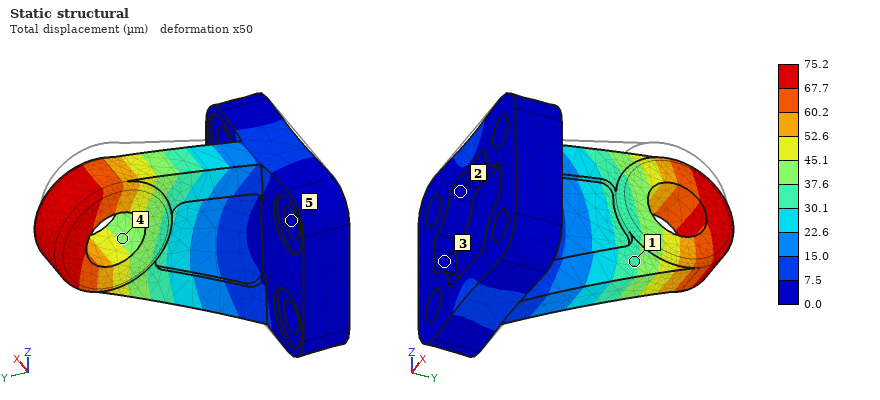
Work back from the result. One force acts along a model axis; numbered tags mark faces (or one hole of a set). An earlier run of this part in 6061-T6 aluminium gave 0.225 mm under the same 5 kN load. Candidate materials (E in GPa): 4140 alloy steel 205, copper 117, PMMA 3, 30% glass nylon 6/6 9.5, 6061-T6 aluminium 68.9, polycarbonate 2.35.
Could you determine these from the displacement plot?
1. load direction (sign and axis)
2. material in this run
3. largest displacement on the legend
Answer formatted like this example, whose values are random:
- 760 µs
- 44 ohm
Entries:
- -Z
- 4140 alloy steel
- 75.2 µm
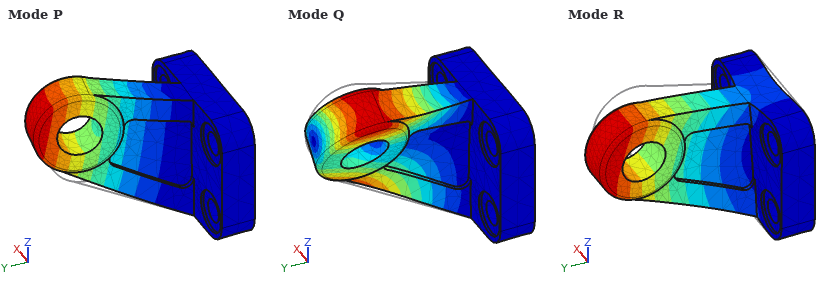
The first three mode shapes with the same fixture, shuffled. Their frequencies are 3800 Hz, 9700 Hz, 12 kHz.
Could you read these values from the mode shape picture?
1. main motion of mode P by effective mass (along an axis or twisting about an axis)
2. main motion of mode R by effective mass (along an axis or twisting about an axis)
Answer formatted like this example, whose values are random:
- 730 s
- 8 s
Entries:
- along X
- along Z
